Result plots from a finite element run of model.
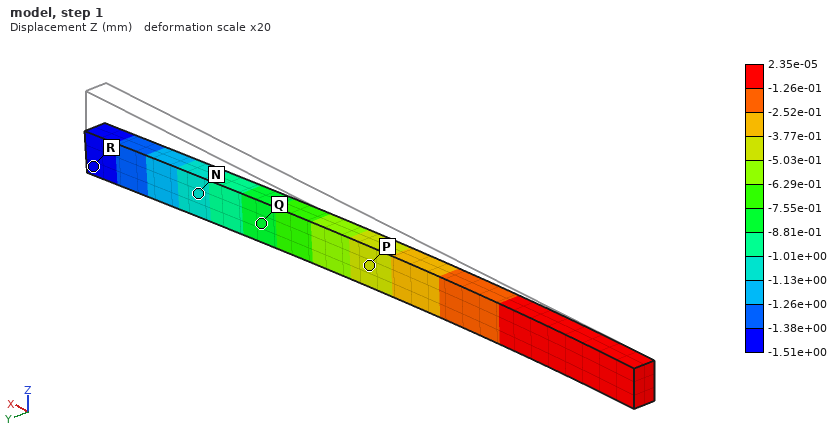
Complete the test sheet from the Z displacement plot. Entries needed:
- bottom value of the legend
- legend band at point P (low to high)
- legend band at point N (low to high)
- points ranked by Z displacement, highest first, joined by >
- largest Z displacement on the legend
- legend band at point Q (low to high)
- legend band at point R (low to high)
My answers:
-1.51e+00 mm
-5.03e-01 to -3.77e-01 mm
-1.13e+00 to -1.01e+00 mm
P > Q > N > R
2.35e-05 mm
-8.81e-01 to -7.55e-01 mm
-1.51e+00 to -1.38e+00 mm
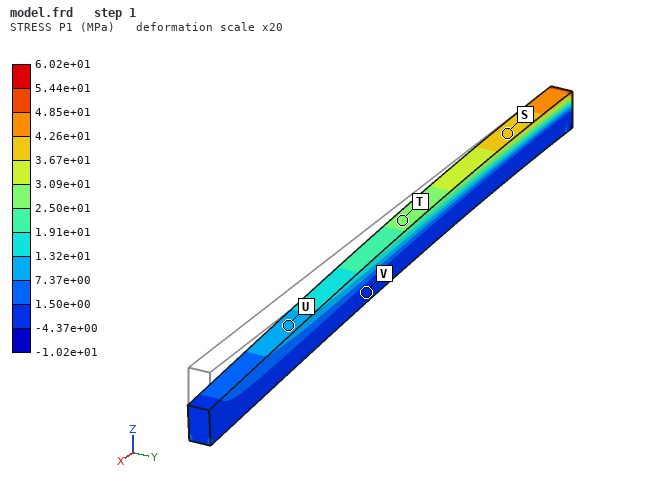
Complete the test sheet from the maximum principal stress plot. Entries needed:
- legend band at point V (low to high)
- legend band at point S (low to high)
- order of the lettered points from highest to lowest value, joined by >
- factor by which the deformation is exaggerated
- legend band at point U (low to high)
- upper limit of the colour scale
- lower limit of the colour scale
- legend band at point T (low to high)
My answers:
-4.37e+00 to 1.50e+00 MPa
3.67e+01 to 4.26e+01 MPa
S > T > U > V
20
7.37e+00 to 1.32e+01 MPa
6.02e+01 MPa
-1.02e+01 MPa
2.50e+01 to 3.09e+01 MPa
